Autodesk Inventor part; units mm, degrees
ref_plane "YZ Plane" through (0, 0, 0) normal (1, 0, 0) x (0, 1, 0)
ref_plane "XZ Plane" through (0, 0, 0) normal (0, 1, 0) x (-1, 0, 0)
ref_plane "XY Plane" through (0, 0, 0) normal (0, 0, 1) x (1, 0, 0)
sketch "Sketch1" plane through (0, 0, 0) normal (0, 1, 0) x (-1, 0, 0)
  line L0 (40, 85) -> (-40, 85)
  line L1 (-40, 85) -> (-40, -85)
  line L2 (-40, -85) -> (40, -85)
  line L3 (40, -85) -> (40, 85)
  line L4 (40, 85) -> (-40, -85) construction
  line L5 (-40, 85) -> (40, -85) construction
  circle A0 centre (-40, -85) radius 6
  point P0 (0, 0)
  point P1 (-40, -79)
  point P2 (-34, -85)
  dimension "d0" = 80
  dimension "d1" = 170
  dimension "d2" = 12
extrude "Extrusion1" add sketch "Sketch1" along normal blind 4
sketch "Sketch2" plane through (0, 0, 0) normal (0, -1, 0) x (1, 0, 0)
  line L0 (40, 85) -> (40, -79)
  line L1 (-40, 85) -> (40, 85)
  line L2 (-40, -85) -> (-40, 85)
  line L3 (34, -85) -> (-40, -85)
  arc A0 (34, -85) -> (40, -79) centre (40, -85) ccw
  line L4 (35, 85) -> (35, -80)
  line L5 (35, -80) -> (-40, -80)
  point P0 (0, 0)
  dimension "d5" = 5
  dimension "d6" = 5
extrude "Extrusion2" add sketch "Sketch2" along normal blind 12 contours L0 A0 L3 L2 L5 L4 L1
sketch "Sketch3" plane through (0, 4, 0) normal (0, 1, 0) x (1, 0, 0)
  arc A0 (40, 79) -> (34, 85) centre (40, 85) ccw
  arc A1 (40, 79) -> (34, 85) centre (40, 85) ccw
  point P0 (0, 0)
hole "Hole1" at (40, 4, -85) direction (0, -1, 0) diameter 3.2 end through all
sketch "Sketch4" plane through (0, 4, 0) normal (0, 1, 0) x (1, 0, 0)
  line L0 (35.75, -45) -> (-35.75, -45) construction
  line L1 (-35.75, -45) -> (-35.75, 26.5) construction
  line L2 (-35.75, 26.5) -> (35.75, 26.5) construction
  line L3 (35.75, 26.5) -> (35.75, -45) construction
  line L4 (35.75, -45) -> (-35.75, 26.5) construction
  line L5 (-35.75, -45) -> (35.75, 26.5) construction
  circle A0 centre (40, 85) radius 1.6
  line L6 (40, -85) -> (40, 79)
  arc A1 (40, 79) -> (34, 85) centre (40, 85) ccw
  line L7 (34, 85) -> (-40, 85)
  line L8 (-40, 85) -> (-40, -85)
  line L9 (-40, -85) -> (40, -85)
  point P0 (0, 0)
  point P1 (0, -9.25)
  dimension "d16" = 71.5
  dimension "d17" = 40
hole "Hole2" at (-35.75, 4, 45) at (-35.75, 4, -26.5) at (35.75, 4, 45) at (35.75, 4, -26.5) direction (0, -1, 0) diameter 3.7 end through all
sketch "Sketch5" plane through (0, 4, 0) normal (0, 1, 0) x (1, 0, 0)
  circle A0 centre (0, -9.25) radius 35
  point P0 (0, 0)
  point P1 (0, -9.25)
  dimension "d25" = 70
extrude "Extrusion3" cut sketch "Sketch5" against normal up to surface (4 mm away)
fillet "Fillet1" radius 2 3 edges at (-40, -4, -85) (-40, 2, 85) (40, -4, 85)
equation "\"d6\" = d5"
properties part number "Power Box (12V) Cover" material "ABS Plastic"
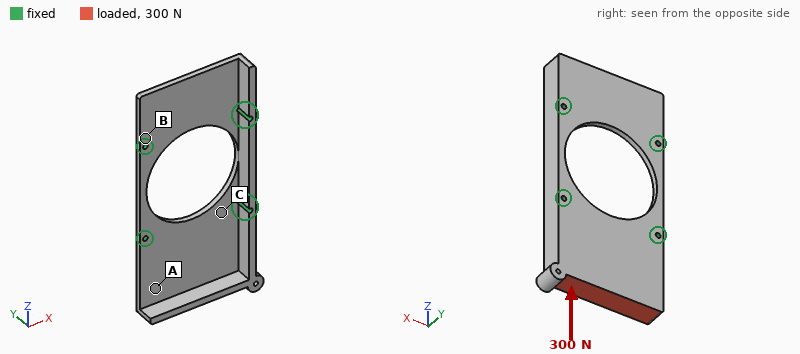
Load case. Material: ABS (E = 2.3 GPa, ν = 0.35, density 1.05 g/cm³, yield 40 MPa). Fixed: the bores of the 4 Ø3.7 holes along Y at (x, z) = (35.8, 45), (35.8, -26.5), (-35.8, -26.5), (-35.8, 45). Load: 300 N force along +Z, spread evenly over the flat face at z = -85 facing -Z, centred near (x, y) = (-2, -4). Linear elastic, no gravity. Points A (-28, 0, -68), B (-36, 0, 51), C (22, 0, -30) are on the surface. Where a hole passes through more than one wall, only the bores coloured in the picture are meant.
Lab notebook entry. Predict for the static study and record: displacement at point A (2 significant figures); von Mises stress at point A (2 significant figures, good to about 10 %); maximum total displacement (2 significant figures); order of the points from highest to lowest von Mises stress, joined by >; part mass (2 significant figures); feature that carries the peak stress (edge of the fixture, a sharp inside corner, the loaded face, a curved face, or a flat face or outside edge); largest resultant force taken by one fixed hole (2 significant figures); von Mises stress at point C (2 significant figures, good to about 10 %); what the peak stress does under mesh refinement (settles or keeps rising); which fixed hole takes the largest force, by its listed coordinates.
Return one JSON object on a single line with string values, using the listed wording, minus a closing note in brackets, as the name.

{"displacement at point A": "0.70 mm", "von Mises stress at point A": "5.5 MPa", "maximum total displacement": "1.7 mm", "order of the points from highest to lowest von Mises stress, joined by >": "A > C > B", "part mass": "57 g", "feature that carries the peak stress": "edge of the fixture", "largest resultant force taken by one fixed hole": "170 N", "von Mises stress at point C": "1.8 MPa", "what the peak stress does under mesh refinement": "keeps rising", "which fixed hole takes the largest force, by its listed coordinates": "(-35.8, -26.5)"}
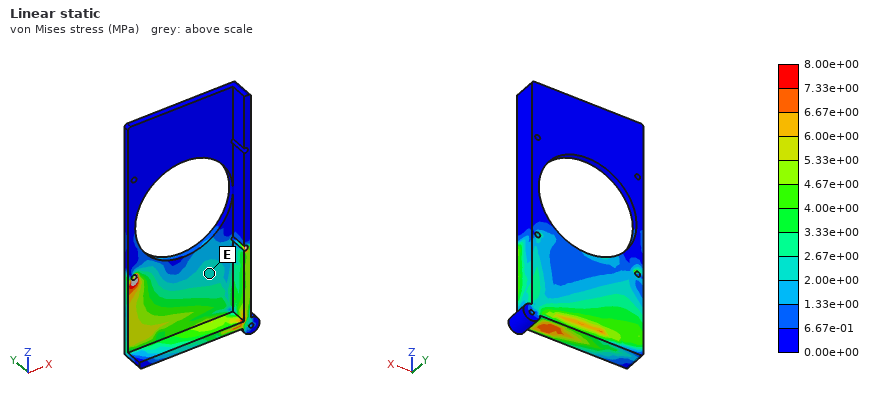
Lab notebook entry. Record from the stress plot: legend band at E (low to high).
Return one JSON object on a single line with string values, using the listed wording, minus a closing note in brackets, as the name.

{"legend band at E": "2.00e+00 to 2.67e+00 MPa"}
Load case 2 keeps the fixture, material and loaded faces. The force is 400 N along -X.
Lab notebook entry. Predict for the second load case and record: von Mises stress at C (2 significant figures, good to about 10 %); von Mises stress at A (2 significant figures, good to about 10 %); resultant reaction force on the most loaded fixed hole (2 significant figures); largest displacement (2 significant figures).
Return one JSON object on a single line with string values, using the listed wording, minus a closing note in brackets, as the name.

{"von Mises stress at C": "3.9 MPa", "von Mises stress at A": "6.4 MPa", "resultant reaction force on the most loaded fixed hole": "380 N", "largest displacement": "2.1 mm"}
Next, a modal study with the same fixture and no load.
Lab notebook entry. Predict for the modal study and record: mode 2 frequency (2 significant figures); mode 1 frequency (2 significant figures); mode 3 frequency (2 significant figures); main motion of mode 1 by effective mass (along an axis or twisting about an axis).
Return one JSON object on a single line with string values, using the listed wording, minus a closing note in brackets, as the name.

{"mode 2 frequency": "550 Hz", "mode 1 frequency": "270 Hz", "mode 3 frequency": "700 Hz", "main motion of mode 1 by effective mass": "along Y"}
